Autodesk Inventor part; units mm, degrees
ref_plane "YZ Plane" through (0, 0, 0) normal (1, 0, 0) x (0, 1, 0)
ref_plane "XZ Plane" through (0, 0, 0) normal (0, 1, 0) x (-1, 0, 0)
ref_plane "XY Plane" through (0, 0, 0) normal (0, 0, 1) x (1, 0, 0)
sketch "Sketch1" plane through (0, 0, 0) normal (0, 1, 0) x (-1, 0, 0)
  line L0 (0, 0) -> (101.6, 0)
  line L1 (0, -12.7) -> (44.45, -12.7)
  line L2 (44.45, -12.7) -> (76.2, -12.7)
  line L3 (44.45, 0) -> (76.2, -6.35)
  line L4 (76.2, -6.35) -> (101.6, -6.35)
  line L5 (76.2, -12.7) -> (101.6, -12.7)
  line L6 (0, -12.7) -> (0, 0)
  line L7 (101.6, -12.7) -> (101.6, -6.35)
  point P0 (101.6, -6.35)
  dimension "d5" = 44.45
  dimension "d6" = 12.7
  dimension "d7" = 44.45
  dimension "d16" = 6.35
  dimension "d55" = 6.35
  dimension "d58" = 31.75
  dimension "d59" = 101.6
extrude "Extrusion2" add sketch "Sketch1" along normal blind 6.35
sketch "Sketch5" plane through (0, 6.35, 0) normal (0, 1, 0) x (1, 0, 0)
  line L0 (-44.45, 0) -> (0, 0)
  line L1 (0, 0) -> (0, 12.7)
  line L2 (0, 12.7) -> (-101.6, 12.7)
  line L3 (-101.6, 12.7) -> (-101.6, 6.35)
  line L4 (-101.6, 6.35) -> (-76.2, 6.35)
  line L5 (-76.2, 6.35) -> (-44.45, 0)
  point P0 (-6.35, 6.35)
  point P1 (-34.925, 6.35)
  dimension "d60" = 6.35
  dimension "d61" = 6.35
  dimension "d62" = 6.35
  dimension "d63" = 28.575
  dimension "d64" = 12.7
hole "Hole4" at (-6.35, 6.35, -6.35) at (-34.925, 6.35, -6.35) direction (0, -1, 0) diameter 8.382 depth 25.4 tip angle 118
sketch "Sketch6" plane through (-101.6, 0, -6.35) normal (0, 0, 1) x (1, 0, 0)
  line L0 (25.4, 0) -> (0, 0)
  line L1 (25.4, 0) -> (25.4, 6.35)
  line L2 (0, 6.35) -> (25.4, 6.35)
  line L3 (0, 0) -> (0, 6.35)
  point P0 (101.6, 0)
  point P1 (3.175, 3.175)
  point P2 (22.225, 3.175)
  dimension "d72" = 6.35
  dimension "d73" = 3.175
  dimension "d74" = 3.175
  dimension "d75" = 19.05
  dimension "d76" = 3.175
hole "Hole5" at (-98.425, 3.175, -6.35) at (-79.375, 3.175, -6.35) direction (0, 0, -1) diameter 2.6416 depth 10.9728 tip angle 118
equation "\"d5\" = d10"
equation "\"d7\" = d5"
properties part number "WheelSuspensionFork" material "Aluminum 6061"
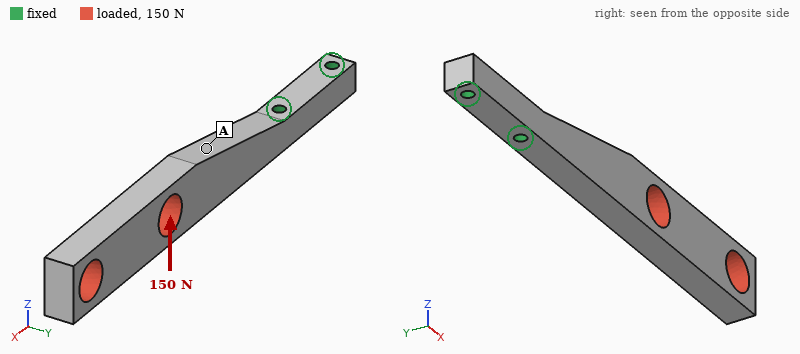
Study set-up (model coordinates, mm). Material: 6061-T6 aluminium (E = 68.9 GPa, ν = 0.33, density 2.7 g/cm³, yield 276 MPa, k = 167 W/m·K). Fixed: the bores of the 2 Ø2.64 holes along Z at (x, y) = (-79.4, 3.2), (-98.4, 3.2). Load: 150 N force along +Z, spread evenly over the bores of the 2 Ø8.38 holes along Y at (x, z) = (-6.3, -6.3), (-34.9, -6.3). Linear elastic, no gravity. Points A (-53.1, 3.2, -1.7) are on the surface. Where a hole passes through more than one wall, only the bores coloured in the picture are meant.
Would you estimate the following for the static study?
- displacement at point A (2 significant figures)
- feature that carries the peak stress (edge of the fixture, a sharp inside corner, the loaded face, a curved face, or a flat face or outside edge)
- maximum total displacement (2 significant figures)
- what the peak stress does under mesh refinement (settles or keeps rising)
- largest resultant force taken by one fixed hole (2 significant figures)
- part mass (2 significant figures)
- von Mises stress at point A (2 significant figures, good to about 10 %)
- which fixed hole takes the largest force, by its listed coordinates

0.21 mm
edge of the fixture
0.84 mm
keeps rising
180 N
16 g
36 MPa
(-79.4, 3.2)
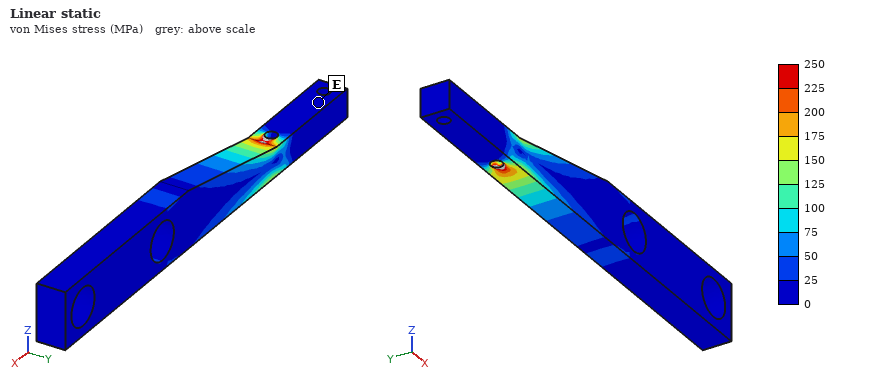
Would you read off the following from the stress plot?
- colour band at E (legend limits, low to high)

0 to 25 MPa
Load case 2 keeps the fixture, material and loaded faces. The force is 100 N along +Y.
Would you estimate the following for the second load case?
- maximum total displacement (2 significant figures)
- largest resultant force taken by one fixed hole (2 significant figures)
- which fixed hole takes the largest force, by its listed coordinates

0.97 mm
190 N
(-79.4, 3.2)
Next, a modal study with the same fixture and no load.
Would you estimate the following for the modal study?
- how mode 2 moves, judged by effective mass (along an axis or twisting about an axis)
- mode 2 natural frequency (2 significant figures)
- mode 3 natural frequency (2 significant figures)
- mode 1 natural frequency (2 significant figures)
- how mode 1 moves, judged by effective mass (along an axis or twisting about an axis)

along Z
890 Hz
4200 Hz
700 Hz
along Y
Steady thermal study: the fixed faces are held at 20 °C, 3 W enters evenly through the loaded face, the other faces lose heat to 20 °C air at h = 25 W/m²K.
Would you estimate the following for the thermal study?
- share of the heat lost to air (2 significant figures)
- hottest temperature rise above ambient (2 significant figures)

22 %
16 K
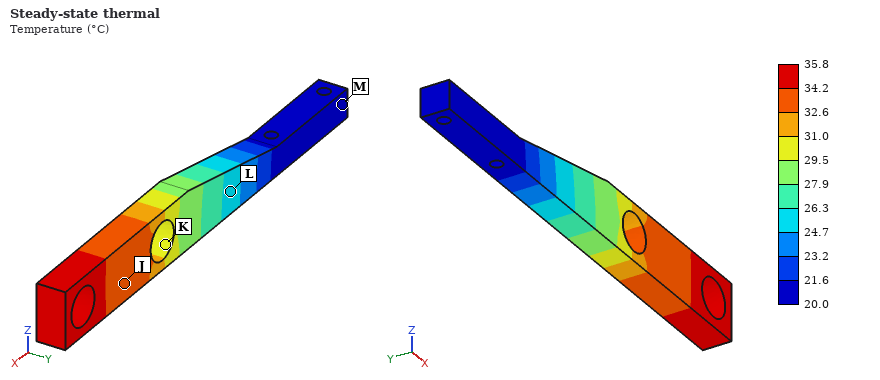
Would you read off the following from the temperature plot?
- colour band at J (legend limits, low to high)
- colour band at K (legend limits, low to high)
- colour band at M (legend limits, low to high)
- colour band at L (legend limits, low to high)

32.6 to 34.2 °C
29.5 to 31.0 °C
20.0 to 21.6 °C
24.7 to 26.3 °C
